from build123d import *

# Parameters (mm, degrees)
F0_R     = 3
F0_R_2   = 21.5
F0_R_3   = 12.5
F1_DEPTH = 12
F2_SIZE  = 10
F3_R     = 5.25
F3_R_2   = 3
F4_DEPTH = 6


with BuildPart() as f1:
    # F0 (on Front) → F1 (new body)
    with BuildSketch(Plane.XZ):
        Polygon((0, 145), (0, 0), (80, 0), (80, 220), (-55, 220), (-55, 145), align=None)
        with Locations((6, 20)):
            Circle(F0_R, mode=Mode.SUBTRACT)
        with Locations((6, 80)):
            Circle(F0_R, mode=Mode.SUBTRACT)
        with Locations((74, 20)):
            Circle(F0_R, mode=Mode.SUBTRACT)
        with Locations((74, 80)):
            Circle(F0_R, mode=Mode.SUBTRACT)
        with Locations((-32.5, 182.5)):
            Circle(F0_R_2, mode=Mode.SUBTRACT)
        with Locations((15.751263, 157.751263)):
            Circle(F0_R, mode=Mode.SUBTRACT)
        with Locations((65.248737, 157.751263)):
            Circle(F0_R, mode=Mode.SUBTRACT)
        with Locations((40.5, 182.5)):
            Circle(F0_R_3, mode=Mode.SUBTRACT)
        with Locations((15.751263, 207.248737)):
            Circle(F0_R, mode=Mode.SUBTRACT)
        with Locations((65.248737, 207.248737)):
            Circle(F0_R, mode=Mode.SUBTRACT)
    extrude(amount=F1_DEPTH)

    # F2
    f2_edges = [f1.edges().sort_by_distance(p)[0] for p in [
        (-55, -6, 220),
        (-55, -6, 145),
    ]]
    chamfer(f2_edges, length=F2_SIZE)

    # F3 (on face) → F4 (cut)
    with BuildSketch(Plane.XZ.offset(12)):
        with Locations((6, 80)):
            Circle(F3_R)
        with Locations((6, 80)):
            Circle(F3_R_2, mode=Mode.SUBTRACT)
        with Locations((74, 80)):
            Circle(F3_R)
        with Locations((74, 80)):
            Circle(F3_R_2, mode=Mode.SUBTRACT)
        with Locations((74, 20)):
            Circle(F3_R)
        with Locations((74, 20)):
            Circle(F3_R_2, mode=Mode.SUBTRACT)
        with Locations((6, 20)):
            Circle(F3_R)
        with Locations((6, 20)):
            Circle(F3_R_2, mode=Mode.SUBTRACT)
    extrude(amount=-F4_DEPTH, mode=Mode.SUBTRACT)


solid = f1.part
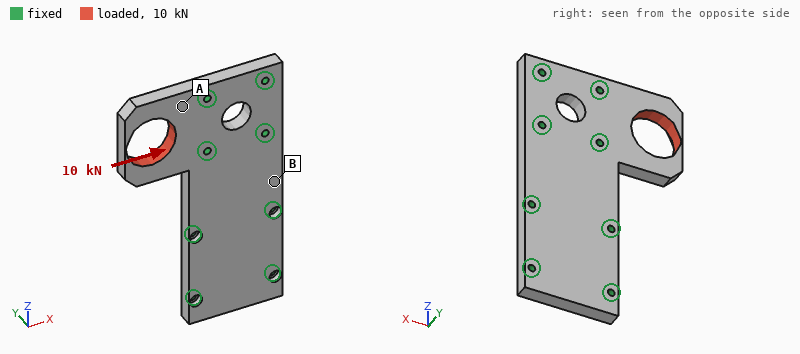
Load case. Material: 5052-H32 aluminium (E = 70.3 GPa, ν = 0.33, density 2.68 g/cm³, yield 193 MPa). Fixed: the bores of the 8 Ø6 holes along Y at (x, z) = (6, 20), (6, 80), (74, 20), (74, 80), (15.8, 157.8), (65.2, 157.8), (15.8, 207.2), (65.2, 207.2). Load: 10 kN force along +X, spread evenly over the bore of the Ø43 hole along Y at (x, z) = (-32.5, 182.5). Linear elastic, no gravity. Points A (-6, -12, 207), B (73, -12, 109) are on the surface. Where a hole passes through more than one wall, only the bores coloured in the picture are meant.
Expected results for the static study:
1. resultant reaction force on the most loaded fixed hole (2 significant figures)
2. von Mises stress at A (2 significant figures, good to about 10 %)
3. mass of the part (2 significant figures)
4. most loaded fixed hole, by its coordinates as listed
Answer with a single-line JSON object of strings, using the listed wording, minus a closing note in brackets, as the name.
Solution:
{"resultant reaction force on the most loaded fixed hole": "4.7 kN", "von Mises stress at A": "17 MPa", "mass of the part": "620 g", "most loaded fixed hole, by its coordinates as listed": "(15.8, 207.2)"}
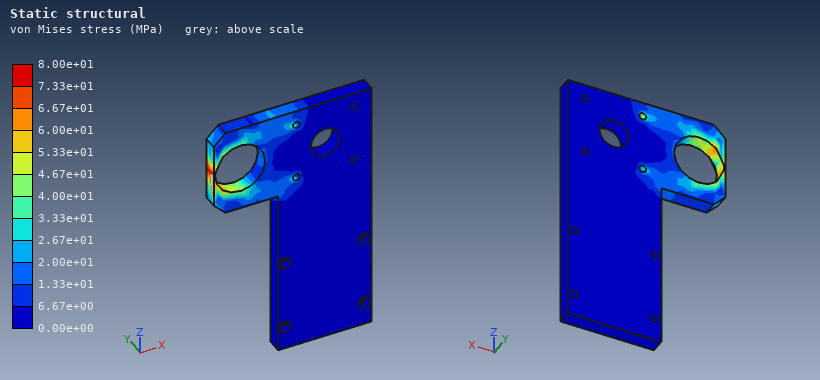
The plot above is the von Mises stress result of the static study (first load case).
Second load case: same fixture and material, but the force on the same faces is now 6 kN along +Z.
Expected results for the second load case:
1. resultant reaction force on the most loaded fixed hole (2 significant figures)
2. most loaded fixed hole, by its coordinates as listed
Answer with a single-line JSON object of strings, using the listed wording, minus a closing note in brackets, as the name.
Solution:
{"resultant reaction force on the most loaded fixed hole": "4.9 kN", "most loaded fixed hole, by its coordinates as listed": "(15.8, 207.2)"}
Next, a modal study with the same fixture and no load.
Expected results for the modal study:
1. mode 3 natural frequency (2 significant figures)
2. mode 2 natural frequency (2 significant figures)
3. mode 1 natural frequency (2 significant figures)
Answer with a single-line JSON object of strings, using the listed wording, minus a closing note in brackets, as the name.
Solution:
{"mode 3 natural frequency": "5900 Hz", "mode 2 natural frequency": "3800 Hz", "mode 1 natural frequency": "2300 Hz"}
